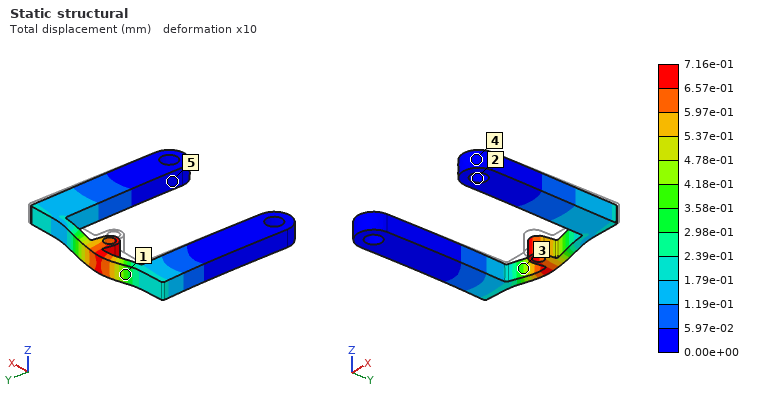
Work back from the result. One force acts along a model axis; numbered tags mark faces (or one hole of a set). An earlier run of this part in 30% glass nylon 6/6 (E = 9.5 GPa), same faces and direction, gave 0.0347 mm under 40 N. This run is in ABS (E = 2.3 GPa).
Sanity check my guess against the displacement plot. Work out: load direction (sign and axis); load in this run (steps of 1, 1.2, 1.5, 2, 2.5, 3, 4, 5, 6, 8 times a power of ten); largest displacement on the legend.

+Y
200 N
7.16e-01 mm
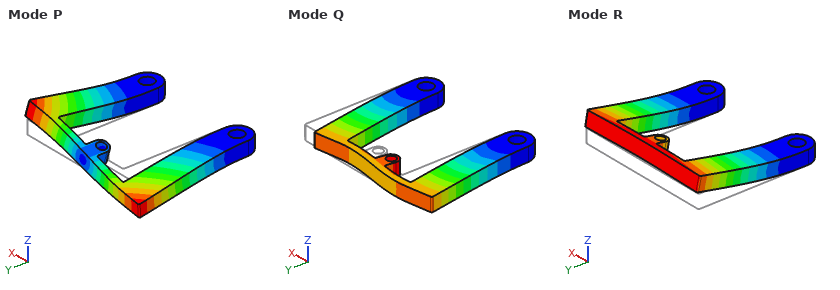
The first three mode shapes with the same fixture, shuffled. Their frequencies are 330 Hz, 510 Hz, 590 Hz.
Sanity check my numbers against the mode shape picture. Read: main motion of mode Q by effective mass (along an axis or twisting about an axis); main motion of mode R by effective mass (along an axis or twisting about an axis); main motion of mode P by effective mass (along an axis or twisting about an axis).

along X
along Z
twisting about Y
